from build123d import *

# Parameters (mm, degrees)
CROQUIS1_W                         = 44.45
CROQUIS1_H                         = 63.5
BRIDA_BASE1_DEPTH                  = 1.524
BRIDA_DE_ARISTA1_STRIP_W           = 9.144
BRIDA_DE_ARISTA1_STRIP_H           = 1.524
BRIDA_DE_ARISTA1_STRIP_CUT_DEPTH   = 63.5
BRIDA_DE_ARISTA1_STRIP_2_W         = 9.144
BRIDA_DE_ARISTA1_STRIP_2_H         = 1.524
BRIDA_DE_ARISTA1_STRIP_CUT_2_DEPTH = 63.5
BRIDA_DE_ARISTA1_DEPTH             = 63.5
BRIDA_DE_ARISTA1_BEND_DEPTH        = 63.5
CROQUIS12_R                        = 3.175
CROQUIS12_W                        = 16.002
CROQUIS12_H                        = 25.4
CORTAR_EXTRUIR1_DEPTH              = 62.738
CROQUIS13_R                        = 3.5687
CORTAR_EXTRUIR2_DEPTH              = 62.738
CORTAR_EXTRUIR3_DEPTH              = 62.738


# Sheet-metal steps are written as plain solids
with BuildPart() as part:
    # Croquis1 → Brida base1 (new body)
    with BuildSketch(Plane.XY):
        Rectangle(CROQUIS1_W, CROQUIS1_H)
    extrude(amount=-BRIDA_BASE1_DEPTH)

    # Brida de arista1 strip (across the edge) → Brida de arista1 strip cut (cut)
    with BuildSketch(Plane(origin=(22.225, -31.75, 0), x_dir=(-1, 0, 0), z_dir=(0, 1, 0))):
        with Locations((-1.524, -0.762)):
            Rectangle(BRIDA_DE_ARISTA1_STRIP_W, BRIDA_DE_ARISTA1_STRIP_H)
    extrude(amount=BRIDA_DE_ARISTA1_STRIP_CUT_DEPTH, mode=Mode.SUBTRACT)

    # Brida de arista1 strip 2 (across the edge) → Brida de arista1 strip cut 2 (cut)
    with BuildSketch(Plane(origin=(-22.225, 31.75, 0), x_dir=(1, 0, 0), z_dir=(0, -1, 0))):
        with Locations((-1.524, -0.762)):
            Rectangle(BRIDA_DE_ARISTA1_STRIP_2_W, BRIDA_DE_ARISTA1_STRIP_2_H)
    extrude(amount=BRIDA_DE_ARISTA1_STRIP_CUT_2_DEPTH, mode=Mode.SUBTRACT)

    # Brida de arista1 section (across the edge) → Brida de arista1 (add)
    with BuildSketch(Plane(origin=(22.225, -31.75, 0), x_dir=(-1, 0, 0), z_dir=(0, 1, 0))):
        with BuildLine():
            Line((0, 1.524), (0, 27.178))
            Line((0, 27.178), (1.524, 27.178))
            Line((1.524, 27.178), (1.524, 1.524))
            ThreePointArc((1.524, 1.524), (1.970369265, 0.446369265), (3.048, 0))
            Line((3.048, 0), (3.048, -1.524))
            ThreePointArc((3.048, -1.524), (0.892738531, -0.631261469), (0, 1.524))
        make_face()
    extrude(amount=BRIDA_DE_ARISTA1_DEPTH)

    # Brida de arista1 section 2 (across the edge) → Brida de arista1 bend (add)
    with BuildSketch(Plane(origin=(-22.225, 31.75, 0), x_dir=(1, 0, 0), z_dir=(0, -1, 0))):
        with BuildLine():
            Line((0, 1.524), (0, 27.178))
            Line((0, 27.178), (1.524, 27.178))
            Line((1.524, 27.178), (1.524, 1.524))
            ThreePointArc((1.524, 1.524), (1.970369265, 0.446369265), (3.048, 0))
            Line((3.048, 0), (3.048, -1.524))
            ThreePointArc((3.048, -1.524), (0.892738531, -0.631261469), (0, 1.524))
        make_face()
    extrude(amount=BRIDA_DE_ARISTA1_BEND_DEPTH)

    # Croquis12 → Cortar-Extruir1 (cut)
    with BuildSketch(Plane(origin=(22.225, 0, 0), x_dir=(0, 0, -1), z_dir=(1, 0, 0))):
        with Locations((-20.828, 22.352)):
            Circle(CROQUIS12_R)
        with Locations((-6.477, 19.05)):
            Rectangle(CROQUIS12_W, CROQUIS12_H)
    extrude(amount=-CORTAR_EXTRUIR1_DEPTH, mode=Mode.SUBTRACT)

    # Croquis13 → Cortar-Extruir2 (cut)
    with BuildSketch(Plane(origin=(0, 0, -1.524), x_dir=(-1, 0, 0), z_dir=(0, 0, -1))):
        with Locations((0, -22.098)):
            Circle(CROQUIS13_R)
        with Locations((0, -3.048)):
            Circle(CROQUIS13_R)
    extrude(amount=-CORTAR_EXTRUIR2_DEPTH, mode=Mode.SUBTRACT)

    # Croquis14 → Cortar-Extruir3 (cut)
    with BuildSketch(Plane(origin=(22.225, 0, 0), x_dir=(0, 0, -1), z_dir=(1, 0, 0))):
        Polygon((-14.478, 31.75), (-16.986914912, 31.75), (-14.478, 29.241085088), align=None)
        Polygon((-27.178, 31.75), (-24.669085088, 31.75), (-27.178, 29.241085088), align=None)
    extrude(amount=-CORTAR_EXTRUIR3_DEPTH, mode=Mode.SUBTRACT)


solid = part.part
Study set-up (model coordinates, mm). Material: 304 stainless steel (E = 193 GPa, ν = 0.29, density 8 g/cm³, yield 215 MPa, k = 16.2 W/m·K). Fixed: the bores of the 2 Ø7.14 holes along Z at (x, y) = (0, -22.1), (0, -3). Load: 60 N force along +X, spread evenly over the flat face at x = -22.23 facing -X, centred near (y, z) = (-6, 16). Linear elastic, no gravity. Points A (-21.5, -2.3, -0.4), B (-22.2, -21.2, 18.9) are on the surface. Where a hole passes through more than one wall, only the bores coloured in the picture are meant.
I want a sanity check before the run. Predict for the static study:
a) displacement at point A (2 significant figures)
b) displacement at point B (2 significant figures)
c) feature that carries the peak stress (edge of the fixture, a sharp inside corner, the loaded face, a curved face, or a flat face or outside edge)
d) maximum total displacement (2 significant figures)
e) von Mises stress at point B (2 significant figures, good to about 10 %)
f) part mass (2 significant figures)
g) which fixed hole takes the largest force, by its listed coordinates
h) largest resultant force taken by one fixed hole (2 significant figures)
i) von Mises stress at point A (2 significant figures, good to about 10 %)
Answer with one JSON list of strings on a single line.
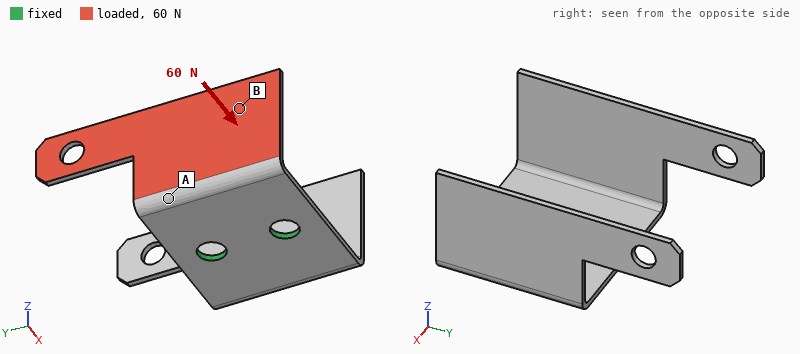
["0.083 mm", "0.21 mm", "a flat face or outside edge", "0.49 mm", "12 MPa", "51 g", "(0, -3)", "48 N", "55 MPa"]
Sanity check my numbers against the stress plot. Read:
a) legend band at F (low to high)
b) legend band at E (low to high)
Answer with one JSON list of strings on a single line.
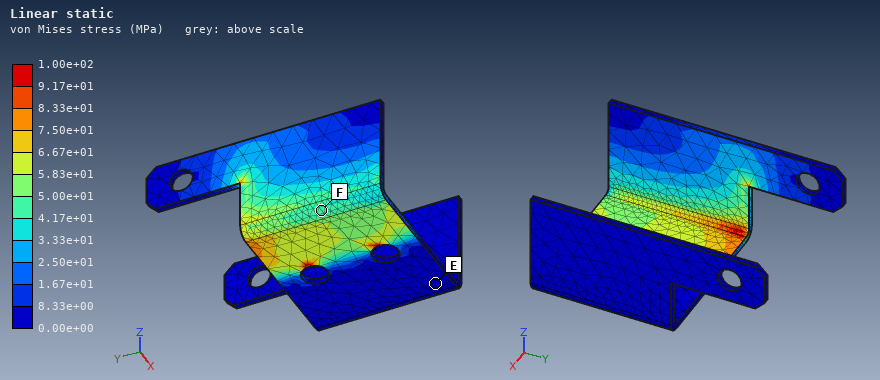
["4.17e+01 to 5.00e+01 MPa", "0.00e+00 to 8.33e+00 MPa"]
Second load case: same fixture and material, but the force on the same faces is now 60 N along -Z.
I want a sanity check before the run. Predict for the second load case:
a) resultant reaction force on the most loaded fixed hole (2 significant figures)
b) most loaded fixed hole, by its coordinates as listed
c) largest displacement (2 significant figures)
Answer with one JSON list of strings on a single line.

["46 N", "(0, -3)", "0.21 mm"]
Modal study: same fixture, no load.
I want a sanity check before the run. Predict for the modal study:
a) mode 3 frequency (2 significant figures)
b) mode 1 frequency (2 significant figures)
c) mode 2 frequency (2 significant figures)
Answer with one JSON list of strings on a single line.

["970 Hz", "570 Hz", "570 Hz"]
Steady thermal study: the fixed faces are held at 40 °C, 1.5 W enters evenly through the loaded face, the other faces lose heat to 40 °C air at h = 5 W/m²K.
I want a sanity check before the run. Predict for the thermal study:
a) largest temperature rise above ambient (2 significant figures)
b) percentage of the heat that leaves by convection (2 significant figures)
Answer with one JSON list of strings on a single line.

["57 K", "28 %"]
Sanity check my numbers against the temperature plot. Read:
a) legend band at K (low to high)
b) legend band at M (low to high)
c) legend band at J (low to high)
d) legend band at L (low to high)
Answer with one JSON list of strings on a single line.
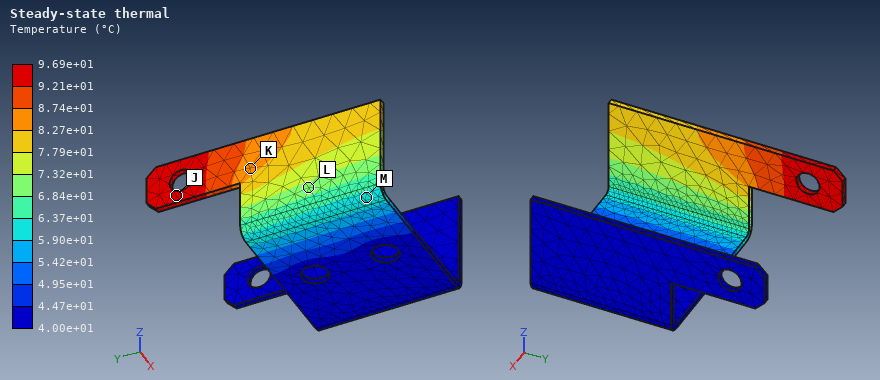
["8.27e+01 to 8.74e+01 °C", "5.90e+01 to 6.37e+01 °C", "9.21e+01 to 9.69e+01 °C", "6.84e+01 to 7.32e+01 °C"]
